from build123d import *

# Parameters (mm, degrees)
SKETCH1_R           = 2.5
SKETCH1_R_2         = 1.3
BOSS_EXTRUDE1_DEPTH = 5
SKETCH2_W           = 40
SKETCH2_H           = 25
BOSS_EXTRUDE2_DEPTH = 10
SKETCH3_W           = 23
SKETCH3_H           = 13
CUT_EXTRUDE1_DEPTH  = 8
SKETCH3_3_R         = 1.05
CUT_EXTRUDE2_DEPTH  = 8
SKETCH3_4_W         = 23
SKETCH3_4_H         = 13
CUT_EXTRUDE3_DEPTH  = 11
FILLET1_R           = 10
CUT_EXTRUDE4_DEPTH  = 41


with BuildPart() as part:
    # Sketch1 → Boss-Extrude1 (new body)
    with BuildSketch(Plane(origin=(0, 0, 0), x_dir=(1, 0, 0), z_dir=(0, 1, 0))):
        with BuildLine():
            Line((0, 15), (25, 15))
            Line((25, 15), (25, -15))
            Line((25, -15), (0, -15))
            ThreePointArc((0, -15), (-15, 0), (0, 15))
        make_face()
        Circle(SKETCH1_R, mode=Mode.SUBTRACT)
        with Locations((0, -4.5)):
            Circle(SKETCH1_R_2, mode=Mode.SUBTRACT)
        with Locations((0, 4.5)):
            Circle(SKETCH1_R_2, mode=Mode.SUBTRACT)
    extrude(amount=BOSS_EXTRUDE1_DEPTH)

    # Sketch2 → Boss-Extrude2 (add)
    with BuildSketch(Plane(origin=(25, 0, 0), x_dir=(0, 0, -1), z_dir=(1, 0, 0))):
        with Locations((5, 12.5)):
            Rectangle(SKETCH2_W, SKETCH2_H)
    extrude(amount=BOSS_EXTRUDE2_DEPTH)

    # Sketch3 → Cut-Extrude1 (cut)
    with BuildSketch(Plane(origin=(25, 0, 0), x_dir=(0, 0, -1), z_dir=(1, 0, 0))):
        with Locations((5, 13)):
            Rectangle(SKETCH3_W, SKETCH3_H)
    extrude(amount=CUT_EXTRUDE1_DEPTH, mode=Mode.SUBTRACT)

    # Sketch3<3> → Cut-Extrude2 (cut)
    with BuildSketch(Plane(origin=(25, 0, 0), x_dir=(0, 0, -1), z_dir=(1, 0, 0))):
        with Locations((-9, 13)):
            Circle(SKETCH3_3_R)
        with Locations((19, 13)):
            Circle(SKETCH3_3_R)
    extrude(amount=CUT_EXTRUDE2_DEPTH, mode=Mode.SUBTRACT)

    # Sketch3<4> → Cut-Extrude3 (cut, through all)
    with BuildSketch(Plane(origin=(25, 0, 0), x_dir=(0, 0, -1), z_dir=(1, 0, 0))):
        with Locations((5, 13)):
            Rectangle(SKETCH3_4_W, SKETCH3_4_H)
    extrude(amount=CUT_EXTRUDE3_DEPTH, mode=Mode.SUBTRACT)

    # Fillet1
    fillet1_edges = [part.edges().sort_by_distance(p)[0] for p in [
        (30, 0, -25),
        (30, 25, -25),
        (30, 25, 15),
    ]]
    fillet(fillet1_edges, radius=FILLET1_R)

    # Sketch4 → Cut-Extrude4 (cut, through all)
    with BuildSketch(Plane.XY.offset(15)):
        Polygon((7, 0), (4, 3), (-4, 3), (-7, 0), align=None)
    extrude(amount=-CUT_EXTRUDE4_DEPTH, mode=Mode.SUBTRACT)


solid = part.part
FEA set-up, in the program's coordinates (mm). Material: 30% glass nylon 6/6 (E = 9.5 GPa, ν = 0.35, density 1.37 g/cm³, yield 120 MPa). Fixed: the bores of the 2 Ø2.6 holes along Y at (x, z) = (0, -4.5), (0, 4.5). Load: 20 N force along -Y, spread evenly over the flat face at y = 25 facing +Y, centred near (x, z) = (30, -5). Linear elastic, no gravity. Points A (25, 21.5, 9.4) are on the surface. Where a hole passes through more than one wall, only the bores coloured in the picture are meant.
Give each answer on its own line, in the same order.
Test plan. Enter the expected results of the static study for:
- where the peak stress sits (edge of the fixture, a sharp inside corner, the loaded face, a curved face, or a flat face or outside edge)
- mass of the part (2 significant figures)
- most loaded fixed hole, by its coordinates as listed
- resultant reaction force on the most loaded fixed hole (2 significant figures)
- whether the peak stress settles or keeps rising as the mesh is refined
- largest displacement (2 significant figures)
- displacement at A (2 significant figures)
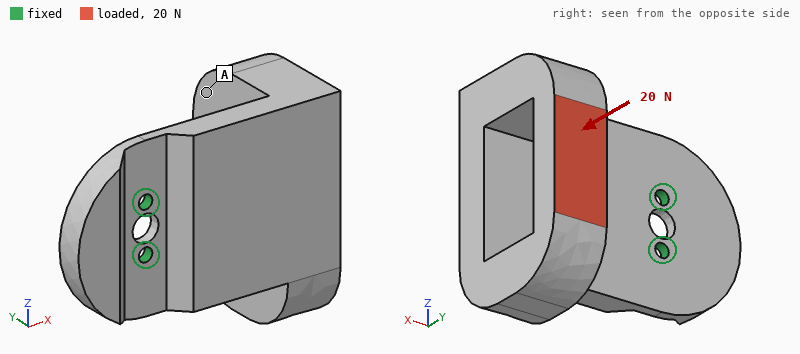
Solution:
edge of the fixture
15 g
(0, -4.5)
18 N
keeps rising
0.70 mm
0.49 mm
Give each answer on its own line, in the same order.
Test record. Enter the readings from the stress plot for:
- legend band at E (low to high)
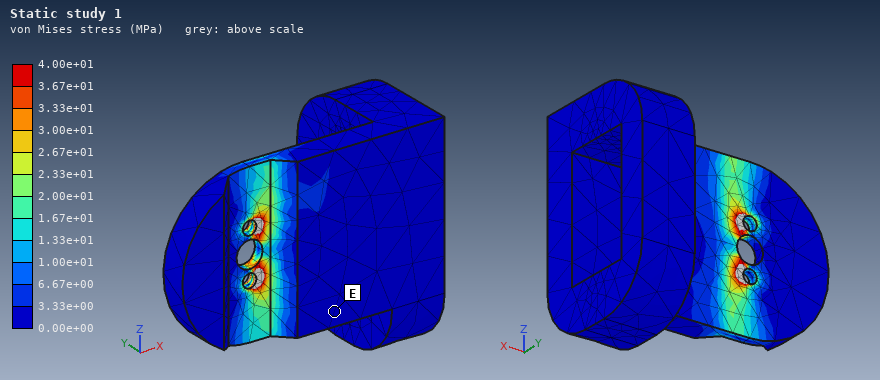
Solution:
0.00e+00 to 3.33e+00 MPa
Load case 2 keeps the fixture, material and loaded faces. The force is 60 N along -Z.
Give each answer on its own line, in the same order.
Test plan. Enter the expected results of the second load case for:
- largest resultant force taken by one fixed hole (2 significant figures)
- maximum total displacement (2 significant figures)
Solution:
190 N
0.49 mm
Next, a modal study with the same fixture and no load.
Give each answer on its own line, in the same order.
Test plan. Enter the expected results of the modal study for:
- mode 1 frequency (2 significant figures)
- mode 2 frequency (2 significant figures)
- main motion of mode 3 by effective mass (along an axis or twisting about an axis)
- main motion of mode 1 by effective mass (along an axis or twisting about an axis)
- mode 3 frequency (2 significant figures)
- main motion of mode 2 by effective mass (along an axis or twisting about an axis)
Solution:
300 Hz
860 Hz
along Z
along Y
2000 Hz
along Z
